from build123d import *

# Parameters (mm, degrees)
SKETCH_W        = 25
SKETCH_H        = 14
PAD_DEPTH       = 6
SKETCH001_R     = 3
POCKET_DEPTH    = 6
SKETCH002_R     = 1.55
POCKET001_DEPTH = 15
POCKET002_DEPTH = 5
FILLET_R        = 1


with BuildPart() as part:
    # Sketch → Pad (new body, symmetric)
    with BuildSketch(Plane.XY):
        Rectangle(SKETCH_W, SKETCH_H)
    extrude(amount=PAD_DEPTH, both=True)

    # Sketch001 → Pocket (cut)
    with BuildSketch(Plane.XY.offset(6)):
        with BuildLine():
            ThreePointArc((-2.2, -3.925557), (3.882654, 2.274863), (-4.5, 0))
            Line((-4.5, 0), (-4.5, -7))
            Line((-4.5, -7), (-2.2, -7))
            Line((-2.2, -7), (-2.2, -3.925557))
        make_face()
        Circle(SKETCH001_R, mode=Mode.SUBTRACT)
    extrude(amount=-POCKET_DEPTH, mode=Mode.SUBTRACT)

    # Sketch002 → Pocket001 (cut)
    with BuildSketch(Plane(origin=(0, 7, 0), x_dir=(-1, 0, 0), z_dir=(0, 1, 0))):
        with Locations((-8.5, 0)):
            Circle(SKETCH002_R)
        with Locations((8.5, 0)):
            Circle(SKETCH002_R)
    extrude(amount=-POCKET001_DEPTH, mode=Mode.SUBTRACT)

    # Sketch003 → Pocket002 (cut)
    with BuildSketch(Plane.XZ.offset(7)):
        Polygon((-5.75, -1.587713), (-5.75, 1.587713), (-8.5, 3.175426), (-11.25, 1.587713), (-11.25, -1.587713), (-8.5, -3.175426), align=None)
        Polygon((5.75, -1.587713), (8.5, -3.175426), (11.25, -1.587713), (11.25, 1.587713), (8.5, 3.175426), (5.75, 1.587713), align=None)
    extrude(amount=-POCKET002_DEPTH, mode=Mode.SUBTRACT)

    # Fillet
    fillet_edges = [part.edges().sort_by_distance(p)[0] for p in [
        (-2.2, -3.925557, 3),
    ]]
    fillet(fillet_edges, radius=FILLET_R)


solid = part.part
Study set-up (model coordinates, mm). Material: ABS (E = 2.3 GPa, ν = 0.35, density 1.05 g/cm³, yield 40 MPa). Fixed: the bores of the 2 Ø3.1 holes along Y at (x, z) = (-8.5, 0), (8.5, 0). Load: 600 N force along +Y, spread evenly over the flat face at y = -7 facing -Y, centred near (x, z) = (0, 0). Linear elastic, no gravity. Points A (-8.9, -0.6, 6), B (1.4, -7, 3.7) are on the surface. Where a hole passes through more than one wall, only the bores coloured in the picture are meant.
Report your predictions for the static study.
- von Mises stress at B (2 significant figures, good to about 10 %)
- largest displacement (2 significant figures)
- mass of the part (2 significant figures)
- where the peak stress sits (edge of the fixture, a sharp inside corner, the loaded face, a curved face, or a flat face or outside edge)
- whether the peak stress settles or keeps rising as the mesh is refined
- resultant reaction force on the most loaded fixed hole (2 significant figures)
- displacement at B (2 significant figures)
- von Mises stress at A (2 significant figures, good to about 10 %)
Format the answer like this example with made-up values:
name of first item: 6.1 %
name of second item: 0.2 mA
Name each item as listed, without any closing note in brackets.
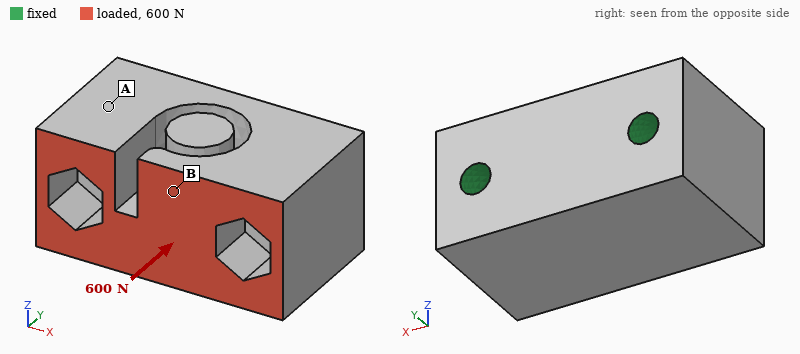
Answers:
von Mises stress at B: 8.3 MPa
largest displacement: 0.13 mm
mass of the part: 3.7 g
where the peak stress sits: a sharp inside corner
whether the peak stress settles or keeps rising as the mesh is refined: keeps rising
resultant reaction force on the most loaded fixed hole: 320 N
displacement at B: 0.067 mm
von Mises stress at A: 1.7 MPa
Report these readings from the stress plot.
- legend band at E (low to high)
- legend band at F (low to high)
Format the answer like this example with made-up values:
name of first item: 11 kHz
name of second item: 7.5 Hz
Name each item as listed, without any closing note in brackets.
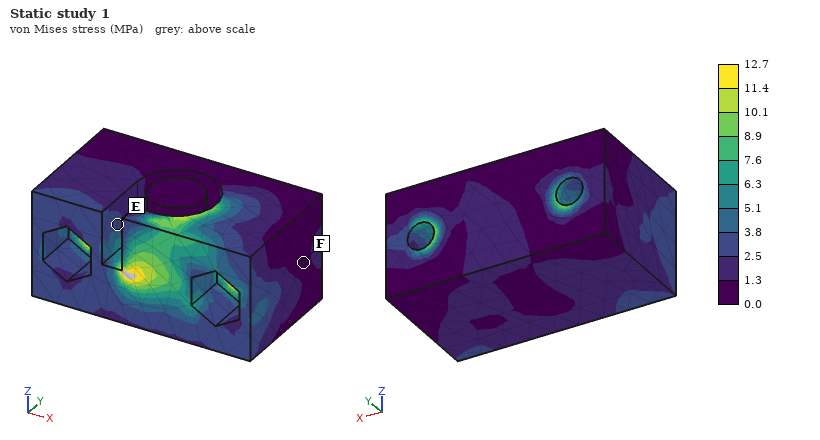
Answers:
legend band at E: 2.5 to 3.8 MPa
legend band at F: 0.0 to 1.3 MPa
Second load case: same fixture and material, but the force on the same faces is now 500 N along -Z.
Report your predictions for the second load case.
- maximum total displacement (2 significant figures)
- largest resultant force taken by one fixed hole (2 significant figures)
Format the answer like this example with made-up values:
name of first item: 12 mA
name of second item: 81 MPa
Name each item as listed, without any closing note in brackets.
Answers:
maximum total displacement: 0.17 mm
largest resultant force taken by one fixed hole: 270 N
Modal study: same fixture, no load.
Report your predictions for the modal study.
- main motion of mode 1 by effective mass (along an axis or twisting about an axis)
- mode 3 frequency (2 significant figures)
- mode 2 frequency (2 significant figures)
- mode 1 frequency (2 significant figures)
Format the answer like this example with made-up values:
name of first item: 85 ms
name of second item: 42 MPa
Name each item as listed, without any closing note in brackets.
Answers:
main motion of mode 1 by effective mass: along Z
mode 3 frequency: 16 kHz
mode 2 frequency: 14 kHz
mode 1 frequency: 12 kHz
